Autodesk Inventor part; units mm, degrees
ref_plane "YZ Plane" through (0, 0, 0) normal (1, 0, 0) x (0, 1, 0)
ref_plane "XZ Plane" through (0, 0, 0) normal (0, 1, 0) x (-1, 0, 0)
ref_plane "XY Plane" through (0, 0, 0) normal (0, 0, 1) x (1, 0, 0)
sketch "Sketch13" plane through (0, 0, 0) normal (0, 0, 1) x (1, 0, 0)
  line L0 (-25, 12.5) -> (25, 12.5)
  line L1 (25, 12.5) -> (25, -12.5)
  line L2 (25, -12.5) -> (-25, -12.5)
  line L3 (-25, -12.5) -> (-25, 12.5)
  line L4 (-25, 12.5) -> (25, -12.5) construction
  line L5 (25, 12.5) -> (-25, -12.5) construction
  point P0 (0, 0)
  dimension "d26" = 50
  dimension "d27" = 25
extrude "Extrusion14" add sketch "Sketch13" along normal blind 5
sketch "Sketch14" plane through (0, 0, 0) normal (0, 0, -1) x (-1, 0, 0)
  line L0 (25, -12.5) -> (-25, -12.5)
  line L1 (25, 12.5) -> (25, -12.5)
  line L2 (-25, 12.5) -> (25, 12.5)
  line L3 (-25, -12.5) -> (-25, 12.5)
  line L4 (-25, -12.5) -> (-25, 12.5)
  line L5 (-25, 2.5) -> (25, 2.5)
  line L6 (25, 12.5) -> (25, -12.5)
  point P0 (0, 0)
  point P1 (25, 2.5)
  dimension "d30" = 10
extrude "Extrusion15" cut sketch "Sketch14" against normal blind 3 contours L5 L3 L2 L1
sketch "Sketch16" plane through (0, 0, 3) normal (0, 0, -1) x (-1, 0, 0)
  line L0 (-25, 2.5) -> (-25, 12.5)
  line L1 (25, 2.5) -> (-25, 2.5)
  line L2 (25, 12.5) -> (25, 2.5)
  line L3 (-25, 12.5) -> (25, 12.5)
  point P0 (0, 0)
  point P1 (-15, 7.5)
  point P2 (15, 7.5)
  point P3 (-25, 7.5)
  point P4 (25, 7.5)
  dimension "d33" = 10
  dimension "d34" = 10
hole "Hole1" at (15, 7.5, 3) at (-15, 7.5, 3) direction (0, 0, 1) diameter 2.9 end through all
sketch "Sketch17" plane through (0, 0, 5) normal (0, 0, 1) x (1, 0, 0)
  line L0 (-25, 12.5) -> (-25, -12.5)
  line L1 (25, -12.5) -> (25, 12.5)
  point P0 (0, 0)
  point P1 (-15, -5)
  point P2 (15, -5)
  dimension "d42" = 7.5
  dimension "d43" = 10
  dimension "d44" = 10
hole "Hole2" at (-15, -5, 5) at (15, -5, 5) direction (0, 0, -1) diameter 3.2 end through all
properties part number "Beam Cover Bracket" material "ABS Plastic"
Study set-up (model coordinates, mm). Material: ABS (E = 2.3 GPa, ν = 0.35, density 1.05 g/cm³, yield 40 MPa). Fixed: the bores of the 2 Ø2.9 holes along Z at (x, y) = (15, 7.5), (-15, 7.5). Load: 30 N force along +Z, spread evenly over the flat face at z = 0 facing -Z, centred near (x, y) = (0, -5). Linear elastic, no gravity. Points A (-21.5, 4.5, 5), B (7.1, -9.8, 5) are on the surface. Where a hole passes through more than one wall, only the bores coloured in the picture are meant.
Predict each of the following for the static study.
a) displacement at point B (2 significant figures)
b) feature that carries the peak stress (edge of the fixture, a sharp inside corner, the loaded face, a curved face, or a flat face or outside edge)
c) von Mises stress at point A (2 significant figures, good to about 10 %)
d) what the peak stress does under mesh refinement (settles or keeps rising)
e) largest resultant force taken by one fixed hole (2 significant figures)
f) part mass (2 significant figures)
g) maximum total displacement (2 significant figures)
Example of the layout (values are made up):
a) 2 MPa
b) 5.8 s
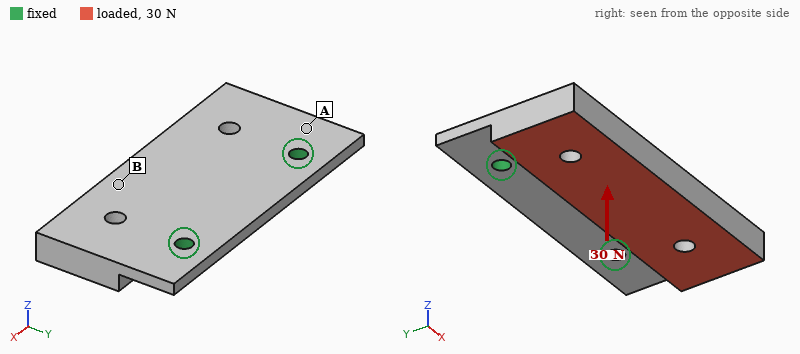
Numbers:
a) 0.43 mm
b) edge of the fixture
c) 6.8 MPa
d) keeps rising
e) 15 N
f) 4.9 g
g) 0.52 mm
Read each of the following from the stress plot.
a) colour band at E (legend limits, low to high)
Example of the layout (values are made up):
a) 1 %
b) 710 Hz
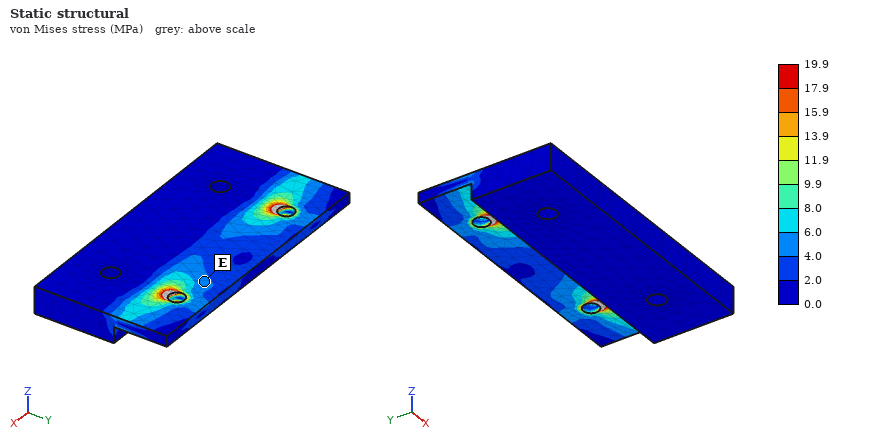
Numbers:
a) 4.0 to 6.0 MPa
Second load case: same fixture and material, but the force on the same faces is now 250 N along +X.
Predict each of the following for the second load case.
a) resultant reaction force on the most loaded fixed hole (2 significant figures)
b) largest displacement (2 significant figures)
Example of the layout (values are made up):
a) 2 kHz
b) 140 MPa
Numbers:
a) 160 N
b) 0.21 mm
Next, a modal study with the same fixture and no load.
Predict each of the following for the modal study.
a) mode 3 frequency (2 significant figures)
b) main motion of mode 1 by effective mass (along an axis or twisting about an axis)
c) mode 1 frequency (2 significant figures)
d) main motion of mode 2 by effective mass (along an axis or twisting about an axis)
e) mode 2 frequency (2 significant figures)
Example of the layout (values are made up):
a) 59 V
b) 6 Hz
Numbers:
a) 3400 Hz
b) along Z
c) 740 Hz
d) twisting about Y
e) 1900 Hz
